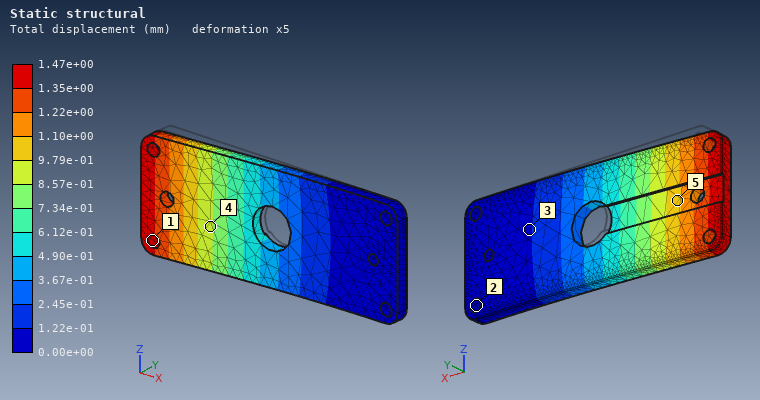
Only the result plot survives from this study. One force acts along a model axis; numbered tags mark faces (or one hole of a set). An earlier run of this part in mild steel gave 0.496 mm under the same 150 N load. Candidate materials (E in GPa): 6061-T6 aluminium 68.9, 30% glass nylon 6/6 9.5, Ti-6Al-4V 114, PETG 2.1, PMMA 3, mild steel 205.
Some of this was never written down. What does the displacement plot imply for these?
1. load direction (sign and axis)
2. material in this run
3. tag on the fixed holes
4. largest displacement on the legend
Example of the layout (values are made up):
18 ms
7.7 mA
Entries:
-Y
6061-T6 aluminium
2
1.47e+00 mm
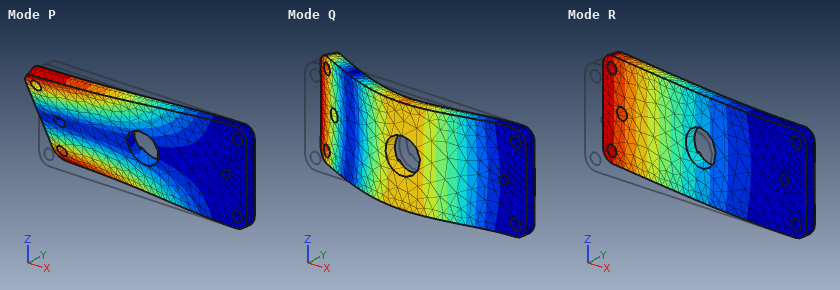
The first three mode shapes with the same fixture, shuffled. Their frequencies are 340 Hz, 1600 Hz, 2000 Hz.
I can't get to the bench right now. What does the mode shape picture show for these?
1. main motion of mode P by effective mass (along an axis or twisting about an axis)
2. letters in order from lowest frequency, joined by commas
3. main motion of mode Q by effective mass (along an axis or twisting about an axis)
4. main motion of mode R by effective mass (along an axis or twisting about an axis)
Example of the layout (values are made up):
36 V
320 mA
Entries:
twisting about X
R, P, Q
along Y
along Y
